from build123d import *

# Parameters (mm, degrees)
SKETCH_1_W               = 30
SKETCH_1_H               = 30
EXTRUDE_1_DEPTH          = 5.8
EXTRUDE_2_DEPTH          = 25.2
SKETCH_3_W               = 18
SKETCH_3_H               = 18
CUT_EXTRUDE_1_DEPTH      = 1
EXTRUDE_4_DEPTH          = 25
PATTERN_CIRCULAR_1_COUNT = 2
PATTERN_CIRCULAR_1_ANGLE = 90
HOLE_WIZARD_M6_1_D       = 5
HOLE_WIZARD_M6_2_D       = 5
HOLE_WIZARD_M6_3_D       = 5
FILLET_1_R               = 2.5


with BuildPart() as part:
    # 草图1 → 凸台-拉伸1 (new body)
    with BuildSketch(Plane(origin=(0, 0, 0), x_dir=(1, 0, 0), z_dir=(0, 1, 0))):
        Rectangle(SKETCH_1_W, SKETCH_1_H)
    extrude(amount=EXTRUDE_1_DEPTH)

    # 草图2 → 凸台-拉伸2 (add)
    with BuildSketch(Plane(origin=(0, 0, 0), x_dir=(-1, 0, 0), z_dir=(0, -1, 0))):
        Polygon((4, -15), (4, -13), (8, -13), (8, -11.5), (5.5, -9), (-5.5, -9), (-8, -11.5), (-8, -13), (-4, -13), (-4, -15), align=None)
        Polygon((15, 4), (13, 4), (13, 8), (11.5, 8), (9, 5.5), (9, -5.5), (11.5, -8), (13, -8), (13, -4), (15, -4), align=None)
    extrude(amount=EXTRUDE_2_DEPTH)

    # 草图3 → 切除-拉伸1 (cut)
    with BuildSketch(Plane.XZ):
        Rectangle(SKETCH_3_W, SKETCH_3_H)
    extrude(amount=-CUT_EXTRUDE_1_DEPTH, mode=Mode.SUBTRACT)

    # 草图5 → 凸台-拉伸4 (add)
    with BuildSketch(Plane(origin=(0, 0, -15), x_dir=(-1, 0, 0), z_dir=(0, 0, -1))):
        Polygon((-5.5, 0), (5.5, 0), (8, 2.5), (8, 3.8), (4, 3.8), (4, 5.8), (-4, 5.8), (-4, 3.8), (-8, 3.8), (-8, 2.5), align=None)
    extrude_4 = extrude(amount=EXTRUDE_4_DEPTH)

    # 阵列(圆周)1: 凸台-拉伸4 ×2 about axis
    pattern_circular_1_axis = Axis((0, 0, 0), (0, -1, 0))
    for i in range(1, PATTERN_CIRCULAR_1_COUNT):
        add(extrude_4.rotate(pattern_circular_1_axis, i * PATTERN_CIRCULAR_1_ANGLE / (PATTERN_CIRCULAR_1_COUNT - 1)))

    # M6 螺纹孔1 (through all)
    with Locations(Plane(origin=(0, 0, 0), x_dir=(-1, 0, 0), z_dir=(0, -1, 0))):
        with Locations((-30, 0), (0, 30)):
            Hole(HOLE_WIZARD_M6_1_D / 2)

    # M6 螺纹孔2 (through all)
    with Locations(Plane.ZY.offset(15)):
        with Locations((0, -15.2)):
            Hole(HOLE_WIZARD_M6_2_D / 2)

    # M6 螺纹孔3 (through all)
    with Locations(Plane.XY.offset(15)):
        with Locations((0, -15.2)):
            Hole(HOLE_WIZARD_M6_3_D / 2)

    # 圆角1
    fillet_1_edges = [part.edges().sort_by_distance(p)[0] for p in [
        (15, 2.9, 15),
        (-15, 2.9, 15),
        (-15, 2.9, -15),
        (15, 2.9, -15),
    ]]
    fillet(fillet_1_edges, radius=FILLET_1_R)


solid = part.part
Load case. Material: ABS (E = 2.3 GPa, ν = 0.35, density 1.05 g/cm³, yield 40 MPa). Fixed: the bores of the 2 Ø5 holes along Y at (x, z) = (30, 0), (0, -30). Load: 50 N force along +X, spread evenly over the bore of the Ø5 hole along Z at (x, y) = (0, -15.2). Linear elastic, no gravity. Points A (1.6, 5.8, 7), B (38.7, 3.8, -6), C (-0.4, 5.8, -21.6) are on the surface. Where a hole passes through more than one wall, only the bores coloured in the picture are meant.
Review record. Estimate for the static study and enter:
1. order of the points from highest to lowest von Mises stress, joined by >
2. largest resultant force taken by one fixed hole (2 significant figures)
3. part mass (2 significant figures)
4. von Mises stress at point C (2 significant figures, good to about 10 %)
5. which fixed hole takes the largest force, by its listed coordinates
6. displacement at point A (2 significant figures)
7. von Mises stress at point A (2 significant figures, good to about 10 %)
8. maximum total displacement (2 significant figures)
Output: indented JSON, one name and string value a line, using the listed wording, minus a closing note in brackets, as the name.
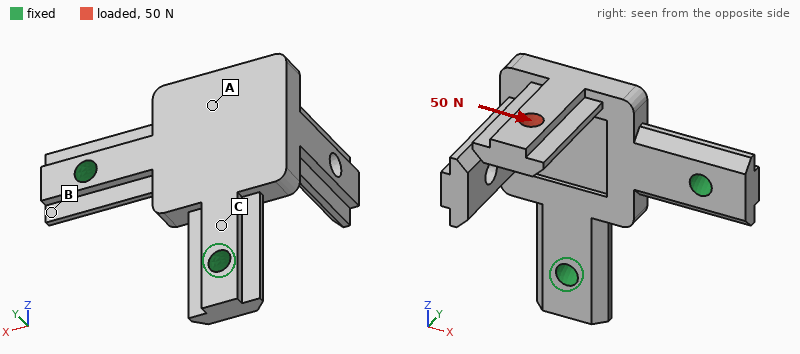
{
  "order of the points from highest to lowest von Mises stress, joined by >": "C > A > B",
  "largest resultant force taken by one fixed hole": "59 N",
  "part mass": "12 g",
  "von Mises stress at point C": "7.5 MPa",
  "which fixed hole takes the largest force, by its listed coordinates": "(30, 0)",
  "displacement at point A": "0.29 mm",
  "von Mises stress at point A": "4.6 MPa",
  "maximum total displacement": "1.0 mm"
}
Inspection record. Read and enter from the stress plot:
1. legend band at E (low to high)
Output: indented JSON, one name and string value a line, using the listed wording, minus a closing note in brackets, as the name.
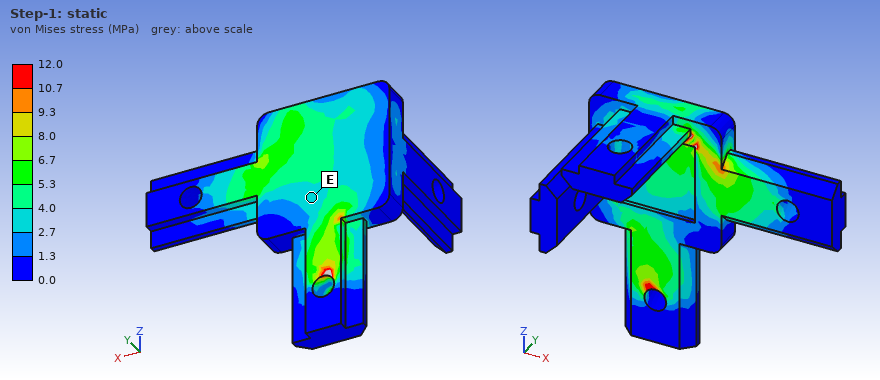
{
  "legend band at E": "2.7 to 4.0 MPa"
}
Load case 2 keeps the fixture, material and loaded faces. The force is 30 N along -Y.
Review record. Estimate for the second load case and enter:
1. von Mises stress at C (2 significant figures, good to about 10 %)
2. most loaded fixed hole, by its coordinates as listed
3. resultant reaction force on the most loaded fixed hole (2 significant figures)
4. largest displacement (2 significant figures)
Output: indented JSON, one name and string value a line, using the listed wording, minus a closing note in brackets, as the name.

{
  "von Mises stress at C": "5.9 MPa",
  "most loaded fixed hole, by its coordinates as listed": "(30, 0)",
  "resultant reaction force on the most loaded fixed hole": "22 N",
  "largest displacement": "0.76 mm"
}
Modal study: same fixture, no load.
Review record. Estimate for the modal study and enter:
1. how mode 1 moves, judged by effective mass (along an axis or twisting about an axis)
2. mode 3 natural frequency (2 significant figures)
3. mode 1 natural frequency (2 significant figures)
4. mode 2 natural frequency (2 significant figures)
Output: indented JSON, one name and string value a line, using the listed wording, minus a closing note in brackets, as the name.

{
  "how mode 1 moves, judged by effective mass": "along Y",
  "mode 3 natural frequency": "1400 Hz",
  "mode 1 natural frequency": "460 Hz",
  "mode 2 natural frequency": "990 Hz"
}
